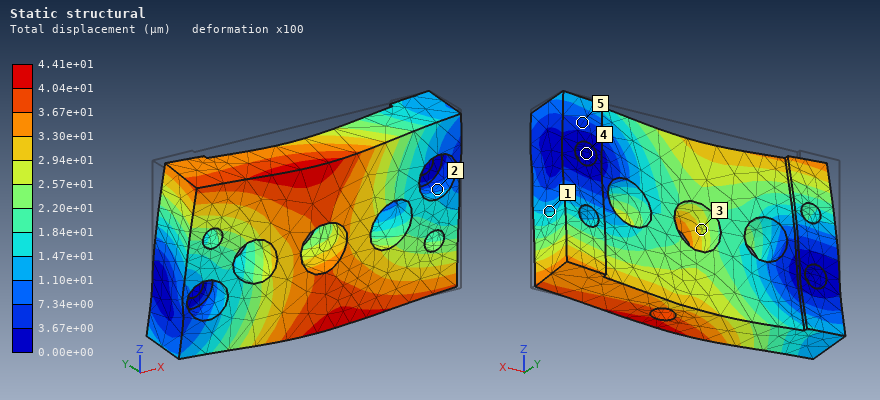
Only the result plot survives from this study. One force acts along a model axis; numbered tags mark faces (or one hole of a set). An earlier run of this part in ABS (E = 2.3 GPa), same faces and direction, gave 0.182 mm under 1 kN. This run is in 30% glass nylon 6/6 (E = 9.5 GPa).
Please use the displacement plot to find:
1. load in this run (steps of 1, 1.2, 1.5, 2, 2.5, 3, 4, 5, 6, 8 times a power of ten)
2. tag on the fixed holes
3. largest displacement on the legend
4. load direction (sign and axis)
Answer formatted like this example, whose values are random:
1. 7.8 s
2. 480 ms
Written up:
1. 1 kN
2. 4
3. 4.41e+01 µm
4. -Z
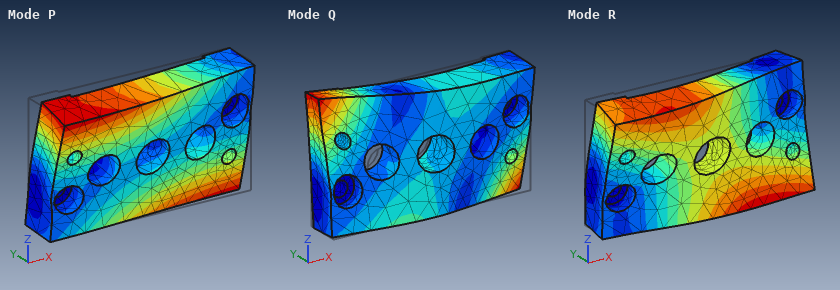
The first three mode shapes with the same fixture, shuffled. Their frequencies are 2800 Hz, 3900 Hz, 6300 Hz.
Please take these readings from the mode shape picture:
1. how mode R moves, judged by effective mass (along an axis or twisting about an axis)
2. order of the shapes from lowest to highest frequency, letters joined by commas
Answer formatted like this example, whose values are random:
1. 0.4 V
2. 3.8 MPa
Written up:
1. along Y
2. P, R, Q
